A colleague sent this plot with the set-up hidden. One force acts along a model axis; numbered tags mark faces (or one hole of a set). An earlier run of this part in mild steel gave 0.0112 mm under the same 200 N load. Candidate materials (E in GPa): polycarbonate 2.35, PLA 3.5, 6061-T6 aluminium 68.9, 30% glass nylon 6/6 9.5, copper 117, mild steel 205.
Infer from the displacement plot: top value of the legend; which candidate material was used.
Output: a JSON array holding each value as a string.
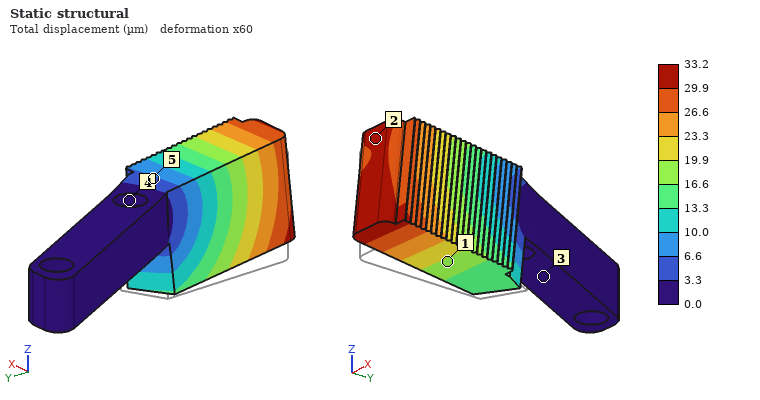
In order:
["33.2 µm", "6061-T6 aluminium"]
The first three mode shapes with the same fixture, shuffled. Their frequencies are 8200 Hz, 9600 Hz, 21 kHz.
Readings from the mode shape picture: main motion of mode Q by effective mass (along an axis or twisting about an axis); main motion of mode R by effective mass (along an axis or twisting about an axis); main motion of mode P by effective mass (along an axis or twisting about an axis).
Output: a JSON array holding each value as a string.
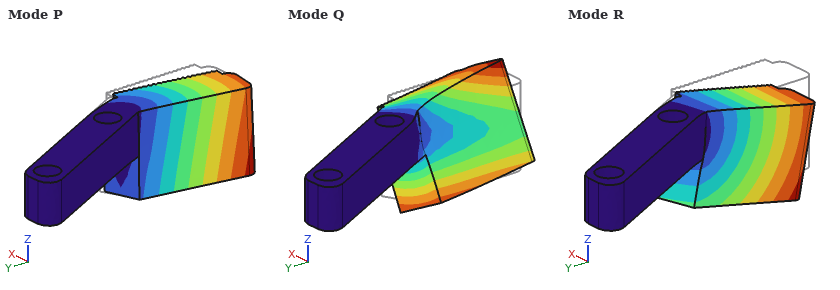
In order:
["twisting about Y", "along Z", "along X"]
